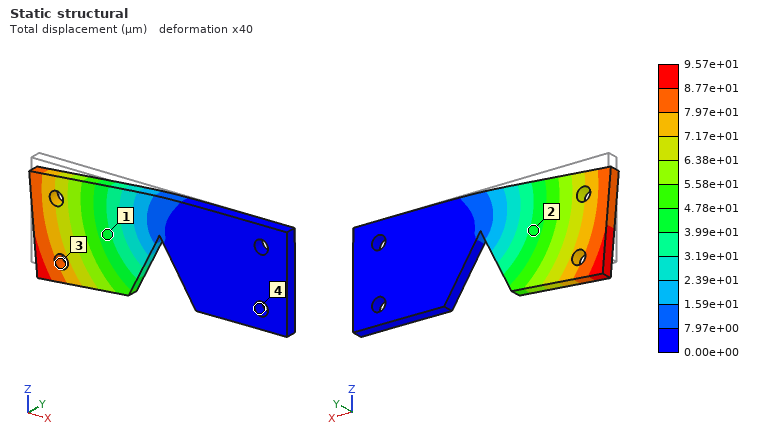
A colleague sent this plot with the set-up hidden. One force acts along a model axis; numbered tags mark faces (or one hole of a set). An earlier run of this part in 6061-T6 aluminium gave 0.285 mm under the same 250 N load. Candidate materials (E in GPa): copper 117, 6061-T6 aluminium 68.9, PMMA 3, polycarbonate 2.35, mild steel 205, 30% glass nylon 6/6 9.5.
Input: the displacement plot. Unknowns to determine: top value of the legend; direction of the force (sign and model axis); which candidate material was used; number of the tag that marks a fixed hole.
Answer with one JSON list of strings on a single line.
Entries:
["9.57e+01 µm", "-Z", "mild steel", "4"]
